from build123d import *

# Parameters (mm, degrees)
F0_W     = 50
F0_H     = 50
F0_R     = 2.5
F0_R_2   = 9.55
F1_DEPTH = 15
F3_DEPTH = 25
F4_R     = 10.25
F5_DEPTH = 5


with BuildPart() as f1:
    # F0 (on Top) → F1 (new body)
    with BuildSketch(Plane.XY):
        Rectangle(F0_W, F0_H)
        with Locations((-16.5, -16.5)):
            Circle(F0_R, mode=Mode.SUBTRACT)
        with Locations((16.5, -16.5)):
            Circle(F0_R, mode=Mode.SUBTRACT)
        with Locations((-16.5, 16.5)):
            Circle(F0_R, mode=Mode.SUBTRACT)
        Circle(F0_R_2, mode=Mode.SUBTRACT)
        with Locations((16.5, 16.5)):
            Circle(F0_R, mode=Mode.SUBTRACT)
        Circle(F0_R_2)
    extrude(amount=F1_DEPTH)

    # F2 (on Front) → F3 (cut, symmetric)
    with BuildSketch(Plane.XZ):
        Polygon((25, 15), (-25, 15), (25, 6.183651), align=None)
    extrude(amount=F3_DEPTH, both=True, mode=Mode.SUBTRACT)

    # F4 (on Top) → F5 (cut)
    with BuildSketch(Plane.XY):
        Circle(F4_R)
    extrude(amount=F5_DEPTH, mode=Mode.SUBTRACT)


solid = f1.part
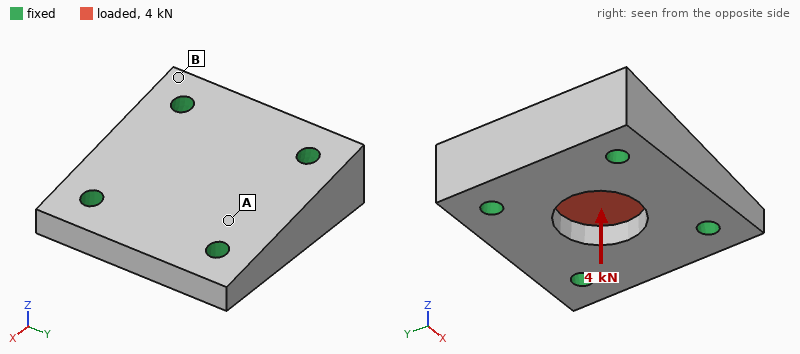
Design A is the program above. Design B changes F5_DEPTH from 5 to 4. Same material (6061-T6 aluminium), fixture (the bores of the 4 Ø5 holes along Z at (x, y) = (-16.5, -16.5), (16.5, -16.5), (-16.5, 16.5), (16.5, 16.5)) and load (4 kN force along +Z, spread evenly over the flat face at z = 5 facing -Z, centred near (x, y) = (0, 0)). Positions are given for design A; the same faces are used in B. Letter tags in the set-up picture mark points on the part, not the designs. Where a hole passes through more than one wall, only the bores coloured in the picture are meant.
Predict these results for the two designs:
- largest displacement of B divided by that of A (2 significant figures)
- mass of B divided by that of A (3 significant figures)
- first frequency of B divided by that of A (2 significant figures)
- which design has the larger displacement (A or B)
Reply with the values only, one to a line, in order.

0.87
1.01
0.98
A
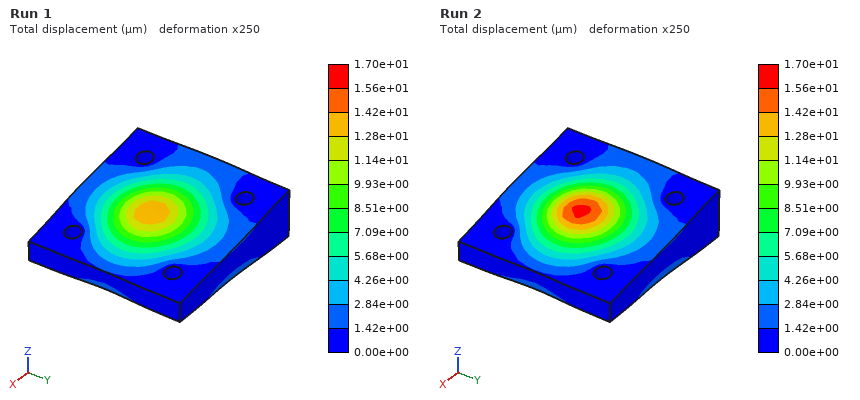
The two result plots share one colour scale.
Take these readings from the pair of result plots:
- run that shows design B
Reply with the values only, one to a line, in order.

Run 1
